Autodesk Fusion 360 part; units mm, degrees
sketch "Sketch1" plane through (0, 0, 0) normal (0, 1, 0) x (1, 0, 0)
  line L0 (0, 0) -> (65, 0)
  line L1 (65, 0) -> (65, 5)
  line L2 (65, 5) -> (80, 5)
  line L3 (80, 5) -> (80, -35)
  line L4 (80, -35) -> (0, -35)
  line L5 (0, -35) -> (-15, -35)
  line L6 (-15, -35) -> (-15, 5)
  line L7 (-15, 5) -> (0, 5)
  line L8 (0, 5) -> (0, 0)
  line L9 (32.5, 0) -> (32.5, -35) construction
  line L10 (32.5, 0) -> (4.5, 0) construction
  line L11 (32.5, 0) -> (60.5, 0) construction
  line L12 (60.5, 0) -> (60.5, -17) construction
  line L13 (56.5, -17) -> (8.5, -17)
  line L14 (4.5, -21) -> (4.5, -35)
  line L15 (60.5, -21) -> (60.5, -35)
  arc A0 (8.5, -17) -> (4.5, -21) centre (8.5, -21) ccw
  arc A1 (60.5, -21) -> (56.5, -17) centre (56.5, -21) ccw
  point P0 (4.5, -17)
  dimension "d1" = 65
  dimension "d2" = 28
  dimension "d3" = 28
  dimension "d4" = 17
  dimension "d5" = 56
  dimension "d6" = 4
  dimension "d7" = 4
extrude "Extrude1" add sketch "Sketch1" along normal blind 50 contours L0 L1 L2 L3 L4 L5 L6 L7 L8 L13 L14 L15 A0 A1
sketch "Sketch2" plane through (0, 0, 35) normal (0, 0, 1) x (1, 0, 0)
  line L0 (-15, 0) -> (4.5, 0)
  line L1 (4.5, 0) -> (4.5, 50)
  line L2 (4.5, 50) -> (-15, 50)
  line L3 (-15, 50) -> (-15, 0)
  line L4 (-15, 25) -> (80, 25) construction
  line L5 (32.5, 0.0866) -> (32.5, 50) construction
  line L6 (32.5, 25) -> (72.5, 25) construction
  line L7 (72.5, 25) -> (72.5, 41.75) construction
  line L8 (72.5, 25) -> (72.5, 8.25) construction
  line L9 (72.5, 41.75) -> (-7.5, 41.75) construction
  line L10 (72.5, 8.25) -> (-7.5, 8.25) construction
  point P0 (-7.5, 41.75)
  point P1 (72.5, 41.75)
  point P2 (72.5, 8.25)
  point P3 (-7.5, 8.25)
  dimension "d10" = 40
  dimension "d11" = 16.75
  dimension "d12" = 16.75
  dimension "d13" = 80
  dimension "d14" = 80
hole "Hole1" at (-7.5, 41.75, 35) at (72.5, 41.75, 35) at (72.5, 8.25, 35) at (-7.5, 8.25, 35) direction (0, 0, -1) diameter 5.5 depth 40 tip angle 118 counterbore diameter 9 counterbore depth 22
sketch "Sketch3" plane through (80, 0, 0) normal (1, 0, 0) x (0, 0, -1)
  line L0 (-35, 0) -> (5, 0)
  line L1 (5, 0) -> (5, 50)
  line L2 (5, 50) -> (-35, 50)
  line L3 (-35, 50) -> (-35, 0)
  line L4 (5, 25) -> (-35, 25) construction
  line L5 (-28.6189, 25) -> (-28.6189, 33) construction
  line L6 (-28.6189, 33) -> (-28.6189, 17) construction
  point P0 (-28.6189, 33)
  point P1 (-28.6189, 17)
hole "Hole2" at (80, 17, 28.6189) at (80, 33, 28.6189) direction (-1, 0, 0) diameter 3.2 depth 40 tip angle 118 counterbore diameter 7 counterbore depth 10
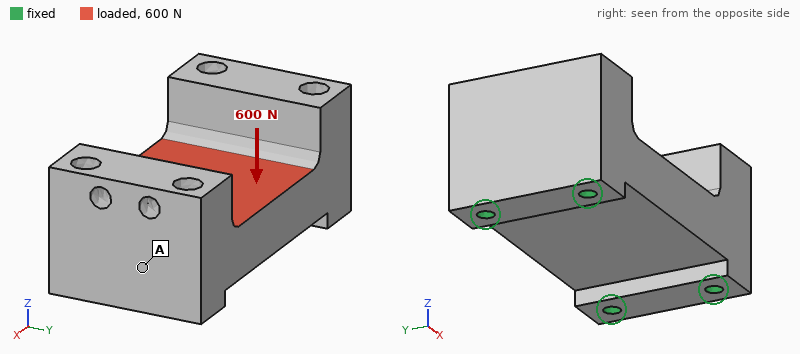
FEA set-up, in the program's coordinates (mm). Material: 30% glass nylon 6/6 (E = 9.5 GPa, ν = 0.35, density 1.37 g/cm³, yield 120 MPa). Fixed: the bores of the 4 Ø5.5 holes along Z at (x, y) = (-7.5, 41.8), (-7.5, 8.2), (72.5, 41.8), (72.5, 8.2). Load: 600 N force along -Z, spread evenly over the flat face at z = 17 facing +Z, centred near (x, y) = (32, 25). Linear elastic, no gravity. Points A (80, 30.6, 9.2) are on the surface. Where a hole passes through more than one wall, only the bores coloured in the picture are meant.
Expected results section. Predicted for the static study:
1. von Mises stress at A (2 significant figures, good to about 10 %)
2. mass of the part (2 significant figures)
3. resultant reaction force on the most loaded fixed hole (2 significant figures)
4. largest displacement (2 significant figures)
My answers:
0.40 MPa
160 g
170 N
11 µm
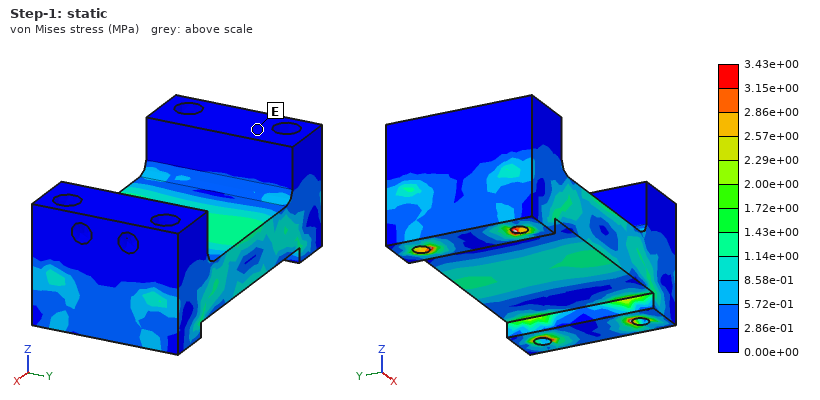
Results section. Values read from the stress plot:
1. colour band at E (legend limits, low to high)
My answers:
0.00e+00 to 2.86e-01 MPa
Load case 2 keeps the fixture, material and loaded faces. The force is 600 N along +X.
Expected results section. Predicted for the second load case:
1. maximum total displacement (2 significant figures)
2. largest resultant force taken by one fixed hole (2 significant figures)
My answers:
1.8 µm
160 N
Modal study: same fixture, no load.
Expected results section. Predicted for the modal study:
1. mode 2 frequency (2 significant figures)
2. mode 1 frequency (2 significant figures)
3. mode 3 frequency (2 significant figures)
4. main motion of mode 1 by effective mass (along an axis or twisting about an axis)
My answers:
7300 Hz
4700 Hz
7500 Hz
along Z
